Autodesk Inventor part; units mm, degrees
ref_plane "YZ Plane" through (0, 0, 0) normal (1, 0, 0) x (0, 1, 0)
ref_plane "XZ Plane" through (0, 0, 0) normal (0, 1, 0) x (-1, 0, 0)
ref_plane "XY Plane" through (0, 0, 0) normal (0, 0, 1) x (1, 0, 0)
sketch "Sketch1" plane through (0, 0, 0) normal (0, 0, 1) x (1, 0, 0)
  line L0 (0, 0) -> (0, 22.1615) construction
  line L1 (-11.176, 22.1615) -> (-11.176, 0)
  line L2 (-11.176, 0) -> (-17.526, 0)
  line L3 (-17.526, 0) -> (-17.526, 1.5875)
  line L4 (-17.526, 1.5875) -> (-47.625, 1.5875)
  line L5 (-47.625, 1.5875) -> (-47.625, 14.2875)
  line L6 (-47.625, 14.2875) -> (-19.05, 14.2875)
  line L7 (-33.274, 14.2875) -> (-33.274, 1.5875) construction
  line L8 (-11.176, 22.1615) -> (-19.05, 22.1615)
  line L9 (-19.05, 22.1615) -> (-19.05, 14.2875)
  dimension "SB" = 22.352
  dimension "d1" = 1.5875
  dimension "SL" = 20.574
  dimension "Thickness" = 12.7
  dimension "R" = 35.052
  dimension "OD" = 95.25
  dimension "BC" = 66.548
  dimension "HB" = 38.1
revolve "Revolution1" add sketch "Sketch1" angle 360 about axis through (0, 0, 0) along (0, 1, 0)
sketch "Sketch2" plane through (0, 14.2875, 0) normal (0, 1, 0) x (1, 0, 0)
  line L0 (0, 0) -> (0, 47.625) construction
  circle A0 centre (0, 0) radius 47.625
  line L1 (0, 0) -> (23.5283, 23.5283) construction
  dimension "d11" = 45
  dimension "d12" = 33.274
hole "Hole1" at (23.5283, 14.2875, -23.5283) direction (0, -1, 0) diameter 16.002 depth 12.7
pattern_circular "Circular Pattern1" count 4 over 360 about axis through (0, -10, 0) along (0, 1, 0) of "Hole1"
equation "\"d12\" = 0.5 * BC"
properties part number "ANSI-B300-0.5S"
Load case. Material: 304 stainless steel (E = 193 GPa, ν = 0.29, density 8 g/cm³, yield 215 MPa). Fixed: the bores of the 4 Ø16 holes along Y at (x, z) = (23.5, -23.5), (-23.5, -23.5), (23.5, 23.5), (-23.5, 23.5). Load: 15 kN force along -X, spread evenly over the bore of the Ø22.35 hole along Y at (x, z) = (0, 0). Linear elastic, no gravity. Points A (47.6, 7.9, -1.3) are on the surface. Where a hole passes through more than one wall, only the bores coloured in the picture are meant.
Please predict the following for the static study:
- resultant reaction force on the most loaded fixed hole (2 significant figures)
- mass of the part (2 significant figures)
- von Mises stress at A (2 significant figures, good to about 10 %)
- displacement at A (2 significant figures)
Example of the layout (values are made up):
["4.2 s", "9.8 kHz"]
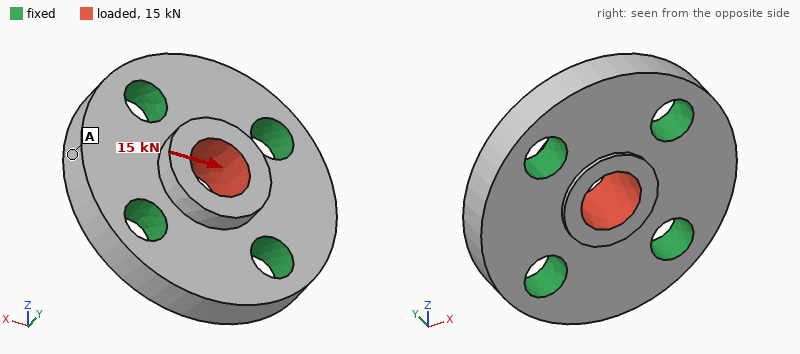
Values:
["4.0 kN", "660 g", "4.6 MPa", "0.61 µm"]
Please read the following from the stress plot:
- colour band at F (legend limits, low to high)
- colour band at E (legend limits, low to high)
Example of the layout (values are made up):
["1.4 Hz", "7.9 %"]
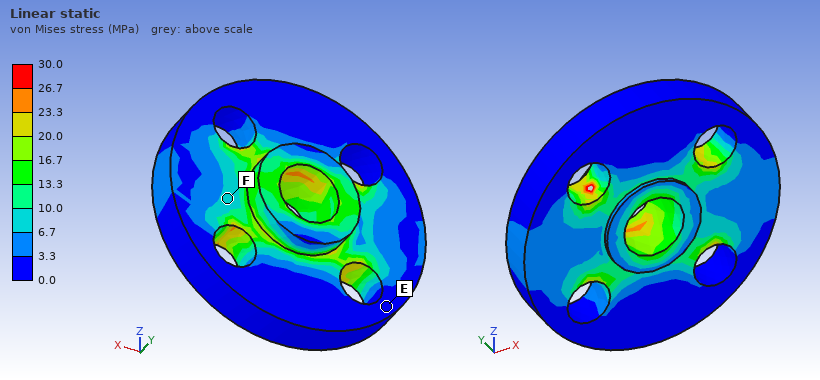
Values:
["6.7 to 10.0 MPa", "0.0 to 3.3 MPa"]
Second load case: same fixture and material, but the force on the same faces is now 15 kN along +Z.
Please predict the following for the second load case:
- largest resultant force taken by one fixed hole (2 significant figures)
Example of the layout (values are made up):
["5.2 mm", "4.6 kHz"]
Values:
["4.0 kN"]
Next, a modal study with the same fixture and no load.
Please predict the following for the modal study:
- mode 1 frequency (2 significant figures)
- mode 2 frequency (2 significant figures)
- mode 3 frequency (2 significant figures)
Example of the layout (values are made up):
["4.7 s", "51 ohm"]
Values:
["20 kHz", "20 kHz", "20 kHz"]
